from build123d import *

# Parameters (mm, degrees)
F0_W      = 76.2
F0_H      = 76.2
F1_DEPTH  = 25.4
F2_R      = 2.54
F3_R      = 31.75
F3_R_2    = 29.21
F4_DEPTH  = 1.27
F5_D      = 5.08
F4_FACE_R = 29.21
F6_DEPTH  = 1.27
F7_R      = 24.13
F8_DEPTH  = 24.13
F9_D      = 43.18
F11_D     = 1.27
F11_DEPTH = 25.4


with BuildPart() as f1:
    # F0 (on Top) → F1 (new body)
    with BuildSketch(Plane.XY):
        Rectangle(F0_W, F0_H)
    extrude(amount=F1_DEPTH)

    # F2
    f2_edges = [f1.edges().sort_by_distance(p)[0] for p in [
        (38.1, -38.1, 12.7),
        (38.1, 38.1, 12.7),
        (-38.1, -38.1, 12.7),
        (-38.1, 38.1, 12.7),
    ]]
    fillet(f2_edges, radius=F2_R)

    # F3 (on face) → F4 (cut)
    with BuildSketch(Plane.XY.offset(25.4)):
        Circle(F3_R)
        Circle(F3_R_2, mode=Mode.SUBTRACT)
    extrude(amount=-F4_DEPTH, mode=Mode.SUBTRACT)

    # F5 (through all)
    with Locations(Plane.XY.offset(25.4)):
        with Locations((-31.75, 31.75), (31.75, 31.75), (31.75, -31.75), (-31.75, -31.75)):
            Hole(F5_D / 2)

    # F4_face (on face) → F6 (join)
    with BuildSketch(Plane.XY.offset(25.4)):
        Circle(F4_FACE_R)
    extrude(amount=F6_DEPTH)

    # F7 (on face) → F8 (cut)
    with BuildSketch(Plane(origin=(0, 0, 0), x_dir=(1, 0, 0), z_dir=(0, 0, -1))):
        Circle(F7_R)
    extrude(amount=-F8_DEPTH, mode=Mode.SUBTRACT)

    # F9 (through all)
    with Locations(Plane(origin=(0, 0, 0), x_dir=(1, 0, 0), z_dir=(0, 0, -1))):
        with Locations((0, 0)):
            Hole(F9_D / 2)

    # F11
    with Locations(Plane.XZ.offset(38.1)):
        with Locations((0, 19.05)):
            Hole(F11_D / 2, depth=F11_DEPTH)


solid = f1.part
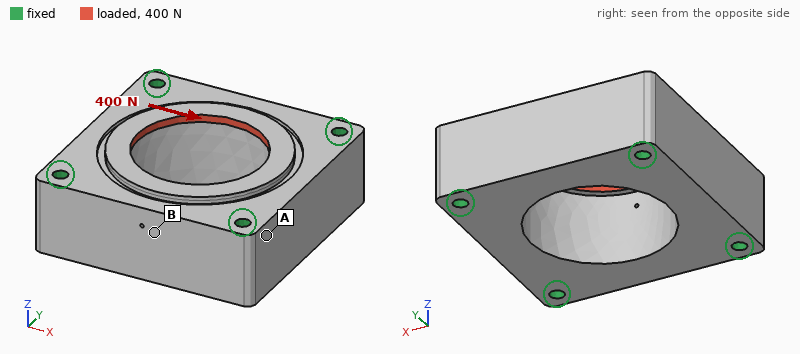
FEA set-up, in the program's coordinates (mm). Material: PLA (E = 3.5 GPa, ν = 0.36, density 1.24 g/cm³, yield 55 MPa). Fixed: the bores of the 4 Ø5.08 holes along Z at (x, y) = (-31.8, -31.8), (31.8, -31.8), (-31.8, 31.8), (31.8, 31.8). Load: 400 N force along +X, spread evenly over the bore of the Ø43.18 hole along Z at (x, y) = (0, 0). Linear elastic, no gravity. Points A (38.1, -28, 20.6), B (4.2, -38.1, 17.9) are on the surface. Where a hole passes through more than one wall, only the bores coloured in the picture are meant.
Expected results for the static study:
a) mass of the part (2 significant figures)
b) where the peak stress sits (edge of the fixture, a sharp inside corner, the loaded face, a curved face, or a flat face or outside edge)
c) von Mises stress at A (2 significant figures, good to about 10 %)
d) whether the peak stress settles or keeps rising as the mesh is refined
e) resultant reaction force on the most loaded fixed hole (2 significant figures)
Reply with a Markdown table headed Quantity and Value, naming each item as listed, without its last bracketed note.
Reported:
| Quantity | Value |
|---|---|
| mass of the part | 120 g |
| where the peak stress sits | a sharp inside corner |
| von Mises stress at A | 0.43 MPa |
| whether the peak stress settles or keeps rising as the mesh is refined | keeps rising |
| resultant reaction force on the most loaded fixed hole | 110 N |
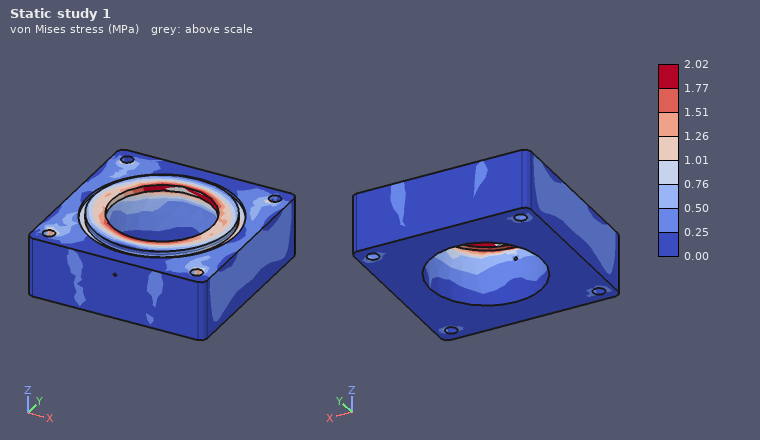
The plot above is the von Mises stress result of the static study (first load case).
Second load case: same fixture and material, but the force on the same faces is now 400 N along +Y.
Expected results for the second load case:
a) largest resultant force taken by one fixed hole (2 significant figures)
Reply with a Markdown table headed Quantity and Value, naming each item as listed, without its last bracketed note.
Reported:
| Quantity | Value |
|---|---|
| largest resultant force taken by one fixed hole | 110 N |
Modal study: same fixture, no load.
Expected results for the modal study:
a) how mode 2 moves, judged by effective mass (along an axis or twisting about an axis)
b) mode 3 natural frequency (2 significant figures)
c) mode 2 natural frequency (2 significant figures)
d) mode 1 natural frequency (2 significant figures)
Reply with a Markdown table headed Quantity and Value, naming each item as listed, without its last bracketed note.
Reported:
| Quantity | Value |
|---|---|
| how mode 2 moves, judged by effective mass | along Z |
| mode 3 natural frequency | 5900 Hz |
| mode 2 natural frequency | 5600 Hz |
| mode 1 natural frequency | 3700 Hz |
